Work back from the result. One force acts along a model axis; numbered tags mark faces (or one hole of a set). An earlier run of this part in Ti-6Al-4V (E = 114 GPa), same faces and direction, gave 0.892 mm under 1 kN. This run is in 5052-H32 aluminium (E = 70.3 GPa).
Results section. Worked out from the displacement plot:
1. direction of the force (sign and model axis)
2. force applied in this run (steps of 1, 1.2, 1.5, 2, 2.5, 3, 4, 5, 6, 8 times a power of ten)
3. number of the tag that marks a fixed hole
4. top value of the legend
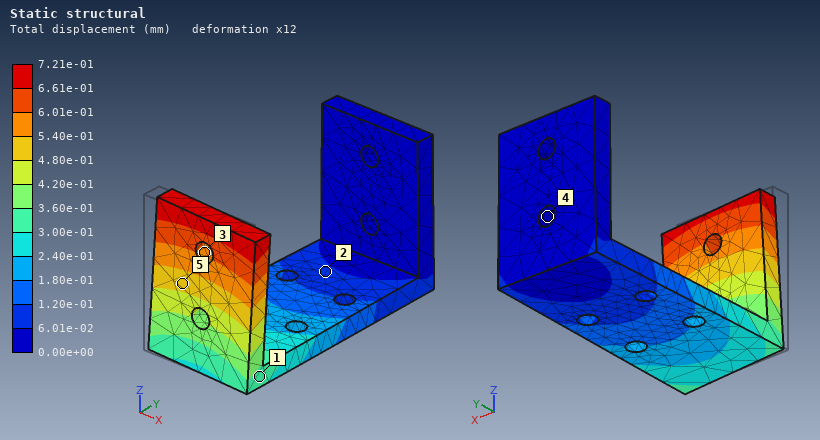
+X
500 N
4
7.21e-01 mm
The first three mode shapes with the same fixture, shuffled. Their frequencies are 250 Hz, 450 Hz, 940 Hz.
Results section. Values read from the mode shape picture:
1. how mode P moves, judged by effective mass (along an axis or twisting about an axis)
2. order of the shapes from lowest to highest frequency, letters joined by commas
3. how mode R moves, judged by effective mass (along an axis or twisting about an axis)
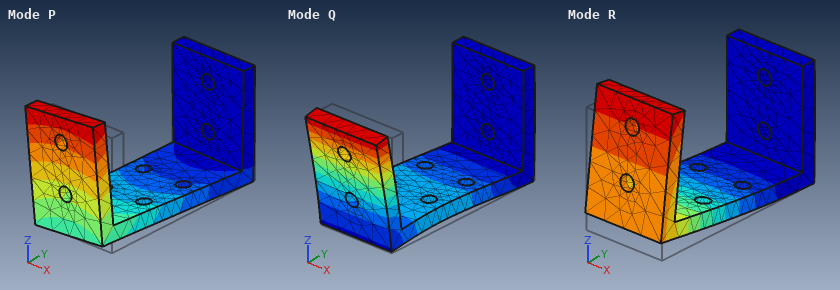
along X
R, P, Q
along Z
